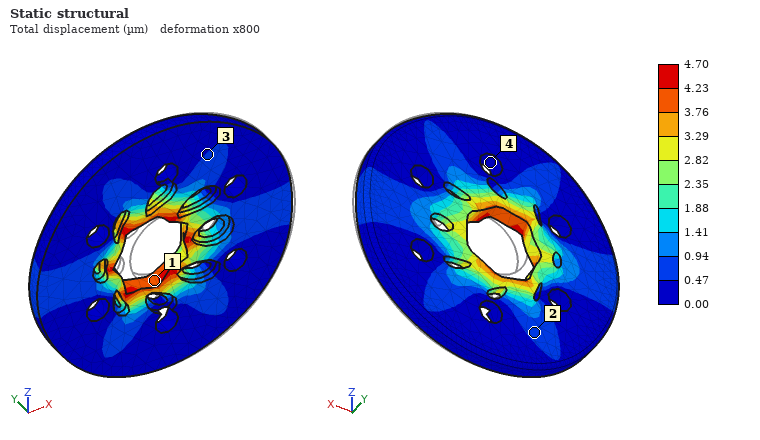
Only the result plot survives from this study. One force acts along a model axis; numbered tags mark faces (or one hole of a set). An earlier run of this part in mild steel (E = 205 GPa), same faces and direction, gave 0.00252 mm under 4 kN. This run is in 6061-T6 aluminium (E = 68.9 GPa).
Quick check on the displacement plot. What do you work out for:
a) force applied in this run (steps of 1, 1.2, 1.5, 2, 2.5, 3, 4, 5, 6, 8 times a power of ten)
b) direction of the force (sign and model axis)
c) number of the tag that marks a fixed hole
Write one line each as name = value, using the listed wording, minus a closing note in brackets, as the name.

force applied in this run = 2.5 kN
direction of the force = -X
number of the tag that marks a fixed hole = 4
